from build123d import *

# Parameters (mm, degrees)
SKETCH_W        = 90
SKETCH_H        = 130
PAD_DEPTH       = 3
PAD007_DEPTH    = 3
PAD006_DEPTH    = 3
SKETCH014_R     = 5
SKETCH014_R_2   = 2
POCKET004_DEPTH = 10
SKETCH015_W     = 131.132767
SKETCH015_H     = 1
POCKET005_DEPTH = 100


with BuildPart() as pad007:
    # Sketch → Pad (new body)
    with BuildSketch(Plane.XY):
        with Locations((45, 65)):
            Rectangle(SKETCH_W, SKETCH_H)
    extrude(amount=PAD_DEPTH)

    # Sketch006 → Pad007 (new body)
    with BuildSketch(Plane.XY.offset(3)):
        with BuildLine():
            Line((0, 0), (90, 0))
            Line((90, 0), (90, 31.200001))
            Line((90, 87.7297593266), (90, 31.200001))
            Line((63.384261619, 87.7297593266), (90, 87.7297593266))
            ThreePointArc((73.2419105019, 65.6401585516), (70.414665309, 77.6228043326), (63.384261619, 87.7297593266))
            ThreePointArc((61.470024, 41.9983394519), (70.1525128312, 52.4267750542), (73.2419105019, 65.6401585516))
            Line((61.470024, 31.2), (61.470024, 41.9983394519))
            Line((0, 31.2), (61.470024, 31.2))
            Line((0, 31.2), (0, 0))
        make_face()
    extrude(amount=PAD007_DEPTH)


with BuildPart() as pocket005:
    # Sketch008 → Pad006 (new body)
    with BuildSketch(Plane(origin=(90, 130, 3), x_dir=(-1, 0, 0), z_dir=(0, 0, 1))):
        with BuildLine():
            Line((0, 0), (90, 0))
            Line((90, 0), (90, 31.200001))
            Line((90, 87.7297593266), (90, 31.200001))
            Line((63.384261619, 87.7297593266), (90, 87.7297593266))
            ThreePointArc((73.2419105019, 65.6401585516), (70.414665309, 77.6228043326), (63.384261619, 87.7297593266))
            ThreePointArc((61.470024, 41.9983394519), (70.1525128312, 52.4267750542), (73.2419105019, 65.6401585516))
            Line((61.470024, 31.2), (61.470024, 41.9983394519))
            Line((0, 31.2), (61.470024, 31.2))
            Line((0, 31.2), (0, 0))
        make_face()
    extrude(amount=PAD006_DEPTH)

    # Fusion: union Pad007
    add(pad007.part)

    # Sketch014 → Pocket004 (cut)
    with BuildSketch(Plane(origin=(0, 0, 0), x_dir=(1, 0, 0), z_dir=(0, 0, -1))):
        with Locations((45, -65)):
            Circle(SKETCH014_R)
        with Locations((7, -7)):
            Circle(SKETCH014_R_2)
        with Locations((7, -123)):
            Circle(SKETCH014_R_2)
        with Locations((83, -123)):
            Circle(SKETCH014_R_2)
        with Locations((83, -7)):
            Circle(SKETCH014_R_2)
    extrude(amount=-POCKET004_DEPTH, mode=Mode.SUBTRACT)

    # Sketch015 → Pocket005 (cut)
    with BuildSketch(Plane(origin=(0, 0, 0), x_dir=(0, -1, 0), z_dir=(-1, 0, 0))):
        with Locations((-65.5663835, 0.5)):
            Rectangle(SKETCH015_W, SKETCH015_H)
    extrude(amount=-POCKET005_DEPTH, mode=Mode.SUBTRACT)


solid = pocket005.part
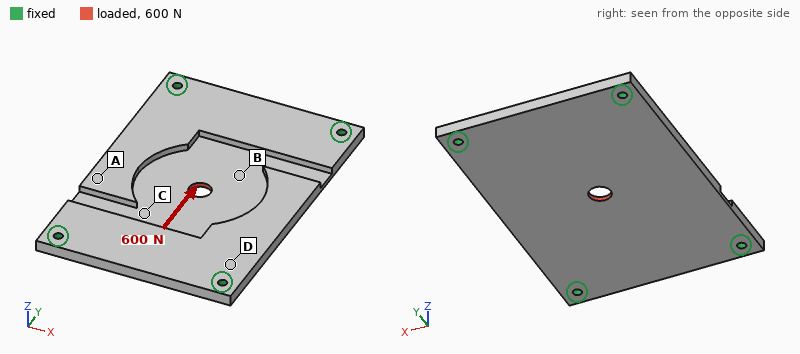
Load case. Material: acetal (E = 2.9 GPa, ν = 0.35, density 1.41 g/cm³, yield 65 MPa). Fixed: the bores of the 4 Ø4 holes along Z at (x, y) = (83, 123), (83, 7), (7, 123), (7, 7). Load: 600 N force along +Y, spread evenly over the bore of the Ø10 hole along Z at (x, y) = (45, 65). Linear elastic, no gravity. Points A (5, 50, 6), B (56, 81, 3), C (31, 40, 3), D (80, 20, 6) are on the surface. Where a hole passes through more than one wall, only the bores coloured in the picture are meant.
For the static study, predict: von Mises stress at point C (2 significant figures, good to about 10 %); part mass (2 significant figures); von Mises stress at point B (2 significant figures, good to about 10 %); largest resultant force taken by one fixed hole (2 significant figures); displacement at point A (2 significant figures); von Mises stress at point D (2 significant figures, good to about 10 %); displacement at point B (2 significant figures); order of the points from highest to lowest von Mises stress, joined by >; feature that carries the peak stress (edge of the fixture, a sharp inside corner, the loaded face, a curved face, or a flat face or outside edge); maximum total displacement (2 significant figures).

3.1 MPa
67 g
4.1 MPa
180 N
31 µm
1.4 MPa
57 µm
B > C > D > A
the loaded face
83 µm
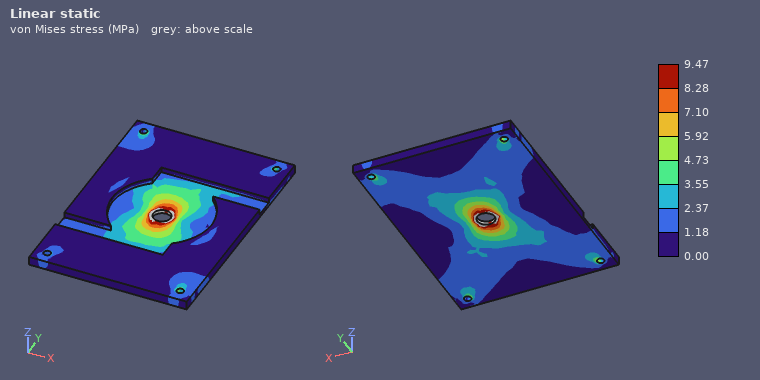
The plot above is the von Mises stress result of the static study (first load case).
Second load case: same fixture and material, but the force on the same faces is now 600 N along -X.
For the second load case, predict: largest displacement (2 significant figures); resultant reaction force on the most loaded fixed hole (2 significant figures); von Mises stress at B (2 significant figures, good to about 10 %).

0.11 mm
200 N
4.3 MPa
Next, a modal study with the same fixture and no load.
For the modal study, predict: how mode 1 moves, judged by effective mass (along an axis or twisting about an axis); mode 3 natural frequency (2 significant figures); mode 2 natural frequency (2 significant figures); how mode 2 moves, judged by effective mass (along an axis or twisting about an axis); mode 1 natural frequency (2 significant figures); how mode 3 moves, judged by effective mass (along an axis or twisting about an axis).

along Z
900 Hz
620 Hz
twisting about Y
450 Hz
twisting about X
